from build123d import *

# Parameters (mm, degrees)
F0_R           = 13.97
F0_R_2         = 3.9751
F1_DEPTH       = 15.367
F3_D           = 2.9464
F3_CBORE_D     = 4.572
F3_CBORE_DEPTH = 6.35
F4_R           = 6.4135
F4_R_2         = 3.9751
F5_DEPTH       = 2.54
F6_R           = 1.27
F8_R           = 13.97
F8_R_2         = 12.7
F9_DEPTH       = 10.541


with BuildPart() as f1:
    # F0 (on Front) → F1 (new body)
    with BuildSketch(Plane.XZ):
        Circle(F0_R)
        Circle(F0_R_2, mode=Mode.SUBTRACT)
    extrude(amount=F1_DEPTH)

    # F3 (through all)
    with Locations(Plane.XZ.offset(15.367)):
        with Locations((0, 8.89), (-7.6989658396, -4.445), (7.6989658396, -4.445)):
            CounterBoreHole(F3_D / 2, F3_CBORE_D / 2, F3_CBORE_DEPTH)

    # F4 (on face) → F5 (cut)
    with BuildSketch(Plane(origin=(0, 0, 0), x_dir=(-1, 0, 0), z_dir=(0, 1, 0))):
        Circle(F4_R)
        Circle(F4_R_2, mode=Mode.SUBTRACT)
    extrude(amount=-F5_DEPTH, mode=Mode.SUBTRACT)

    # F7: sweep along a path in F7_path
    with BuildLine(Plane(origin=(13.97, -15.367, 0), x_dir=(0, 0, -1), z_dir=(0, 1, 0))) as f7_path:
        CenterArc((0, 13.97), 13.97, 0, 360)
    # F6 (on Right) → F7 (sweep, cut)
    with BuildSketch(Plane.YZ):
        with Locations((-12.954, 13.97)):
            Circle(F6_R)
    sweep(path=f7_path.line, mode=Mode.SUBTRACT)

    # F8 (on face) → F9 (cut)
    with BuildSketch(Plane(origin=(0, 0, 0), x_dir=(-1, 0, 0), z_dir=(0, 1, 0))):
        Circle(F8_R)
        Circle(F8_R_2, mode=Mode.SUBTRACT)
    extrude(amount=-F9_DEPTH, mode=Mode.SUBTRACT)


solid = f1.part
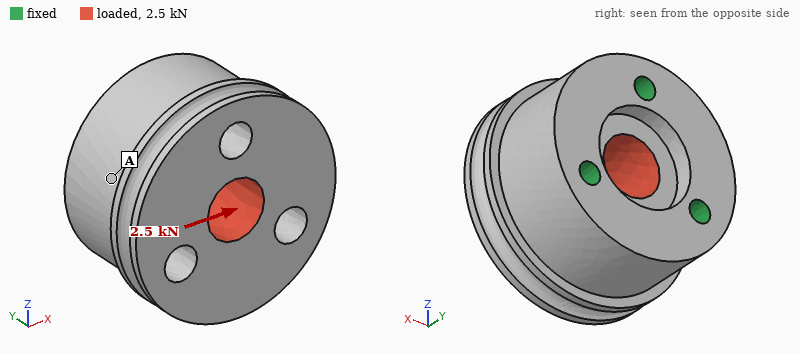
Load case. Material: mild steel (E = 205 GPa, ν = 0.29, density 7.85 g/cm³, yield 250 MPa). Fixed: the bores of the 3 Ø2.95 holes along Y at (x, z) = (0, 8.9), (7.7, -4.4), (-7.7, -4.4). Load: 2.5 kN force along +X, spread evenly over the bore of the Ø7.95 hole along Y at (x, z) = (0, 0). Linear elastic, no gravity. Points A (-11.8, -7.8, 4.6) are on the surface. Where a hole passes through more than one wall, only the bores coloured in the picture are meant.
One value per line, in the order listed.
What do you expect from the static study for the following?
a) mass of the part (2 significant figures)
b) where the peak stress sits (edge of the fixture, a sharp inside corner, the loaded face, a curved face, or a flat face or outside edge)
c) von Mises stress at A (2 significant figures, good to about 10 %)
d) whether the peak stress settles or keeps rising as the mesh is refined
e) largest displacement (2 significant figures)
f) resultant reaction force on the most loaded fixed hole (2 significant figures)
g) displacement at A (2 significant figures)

52 g
edge of the fixture
5.1 MPa
keeps rising
1.1 µm
890 N
0.61 µm
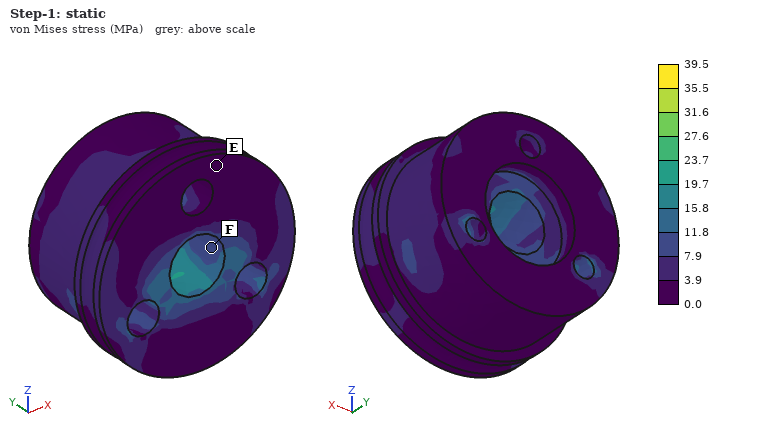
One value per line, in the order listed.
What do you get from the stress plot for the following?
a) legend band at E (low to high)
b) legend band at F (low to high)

0.0 to 3.9 MPa
7.9 to 11.8 MPa
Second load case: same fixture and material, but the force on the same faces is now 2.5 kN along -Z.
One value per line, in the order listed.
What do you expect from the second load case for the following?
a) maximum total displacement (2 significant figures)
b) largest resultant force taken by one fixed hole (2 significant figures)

1.2 µm
900 N
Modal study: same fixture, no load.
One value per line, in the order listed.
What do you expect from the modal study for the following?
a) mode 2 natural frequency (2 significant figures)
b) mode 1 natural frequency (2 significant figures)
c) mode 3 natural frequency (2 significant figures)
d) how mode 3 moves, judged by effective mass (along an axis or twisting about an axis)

42 kHz
42 kHz
60 kHz
along Y
